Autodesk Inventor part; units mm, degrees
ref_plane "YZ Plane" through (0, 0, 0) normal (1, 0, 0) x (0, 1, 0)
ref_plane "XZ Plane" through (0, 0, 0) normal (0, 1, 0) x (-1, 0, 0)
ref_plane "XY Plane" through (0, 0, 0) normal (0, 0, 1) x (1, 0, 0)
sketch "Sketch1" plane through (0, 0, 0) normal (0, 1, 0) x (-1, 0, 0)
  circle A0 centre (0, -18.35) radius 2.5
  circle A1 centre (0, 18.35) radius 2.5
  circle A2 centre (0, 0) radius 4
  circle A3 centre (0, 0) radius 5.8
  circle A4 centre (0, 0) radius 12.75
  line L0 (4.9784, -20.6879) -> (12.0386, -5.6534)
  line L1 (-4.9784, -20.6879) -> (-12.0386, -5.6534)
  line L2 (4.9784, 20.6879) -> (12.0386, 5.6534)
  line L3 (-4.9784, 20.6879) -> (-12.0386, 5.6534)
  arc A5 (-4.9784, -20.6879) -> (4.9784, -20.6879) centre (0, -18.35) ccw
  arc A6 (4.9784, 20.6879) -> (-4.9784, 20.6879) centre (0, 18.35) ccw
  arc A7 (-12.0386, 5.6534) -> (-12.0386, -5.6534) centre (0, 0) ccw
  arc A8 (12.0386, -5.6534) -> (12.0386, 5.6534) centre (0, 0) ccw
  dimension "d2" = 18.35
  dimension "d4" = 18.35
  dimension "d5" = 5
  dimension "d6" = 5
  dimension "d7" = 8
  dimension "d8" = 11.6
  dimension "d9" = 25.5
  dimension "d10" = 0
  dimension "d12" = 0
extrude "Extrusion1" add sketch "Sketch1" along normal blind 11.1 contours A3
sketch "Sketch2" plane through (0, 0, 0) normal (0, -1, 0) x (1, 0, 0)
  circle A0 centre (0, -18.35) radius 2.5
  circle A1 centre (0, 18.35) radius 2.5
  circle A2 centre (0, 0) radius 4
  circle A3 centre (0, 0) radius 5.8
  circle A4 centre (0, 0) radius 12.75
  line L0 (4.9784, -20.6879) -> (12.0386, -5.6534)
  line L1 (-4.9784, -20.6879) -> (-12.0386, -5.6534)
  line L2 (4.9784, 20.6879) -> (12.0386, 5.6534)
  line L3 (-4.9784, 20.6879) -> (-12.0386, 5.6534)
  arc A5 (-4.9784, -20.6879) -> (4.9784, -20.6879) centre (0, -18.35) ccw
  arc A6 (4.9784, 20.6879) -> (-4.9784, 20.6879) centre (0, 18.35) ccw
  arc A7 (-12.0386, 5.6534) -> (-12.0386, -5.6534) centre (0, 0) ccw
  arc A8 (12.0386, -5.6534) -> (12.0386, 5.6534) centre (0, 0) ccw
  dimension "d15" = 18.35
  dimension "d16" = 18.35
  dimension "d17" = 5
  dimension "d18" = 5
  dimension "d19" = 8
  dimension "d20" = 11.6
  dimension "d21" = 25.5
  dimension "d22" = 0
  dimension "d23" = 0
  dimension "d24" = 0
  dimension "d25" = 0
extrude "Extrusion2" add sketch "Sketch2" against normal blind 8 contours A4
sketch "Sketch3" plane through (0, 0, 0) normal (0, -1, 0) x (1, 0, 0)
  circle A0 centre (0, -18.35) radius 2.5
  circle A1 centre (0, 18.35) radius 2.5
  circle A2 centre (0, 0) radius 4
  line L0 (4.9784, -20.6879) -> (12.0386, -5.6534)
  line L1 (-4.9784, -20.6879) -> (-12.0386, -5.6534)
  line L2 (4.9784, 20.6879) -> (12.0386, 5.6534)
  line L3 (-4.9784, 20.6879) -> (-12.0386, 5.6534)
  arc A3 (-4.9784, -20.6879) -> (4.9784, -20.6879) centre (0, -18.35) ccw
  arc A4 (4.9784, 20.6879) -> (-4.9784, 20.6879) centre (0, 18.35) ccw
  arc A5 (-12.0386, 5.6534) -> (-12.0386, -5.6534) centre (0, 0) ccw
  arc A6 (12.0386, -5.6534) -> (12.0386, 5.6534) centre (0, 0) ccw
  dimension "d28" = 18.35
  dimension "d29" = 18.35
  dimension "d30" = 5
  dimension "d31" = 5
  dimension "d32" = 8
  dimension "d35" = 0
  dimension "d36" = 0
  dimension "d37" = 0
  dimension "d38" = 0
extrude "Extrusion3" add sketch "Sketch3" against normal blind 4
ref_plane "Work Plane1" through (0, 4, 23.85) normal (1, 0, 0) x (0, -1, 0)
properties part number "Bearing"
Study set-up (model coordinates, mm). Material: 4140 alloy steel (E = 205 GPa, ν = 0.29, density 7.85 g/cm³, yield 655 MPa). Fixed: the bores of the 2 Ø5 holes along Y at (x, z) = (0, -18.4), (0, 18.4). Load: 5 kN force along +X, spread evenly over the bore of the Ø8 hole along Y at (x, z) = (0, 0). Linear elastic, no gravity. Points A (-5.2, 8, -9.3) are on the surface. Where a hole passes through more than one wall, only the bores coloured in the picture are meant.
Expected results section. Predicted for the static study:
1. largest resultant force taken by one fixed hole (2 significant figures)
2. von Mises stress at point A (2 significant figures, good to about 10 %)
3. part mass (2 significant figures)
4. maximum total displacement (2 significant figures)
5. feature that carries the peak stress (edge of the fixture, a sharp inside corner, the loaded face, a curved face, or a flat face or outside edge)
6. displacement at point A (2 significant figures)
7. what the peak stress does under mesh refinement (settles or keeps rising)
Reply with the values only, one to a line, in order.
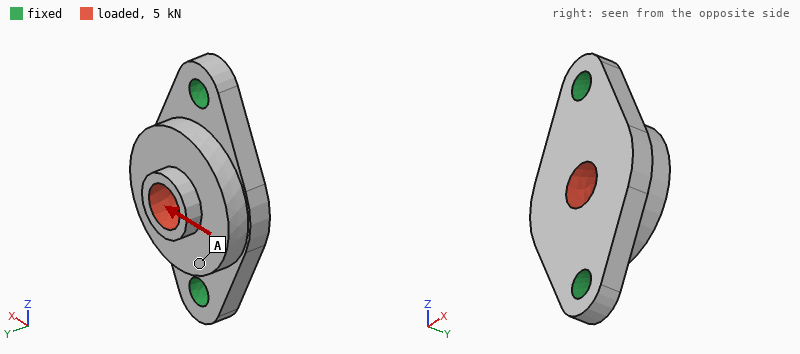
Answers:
2.5 kN
43 MPa
40 g
32 µm
edge of the fixture
20 µm
keeps rising
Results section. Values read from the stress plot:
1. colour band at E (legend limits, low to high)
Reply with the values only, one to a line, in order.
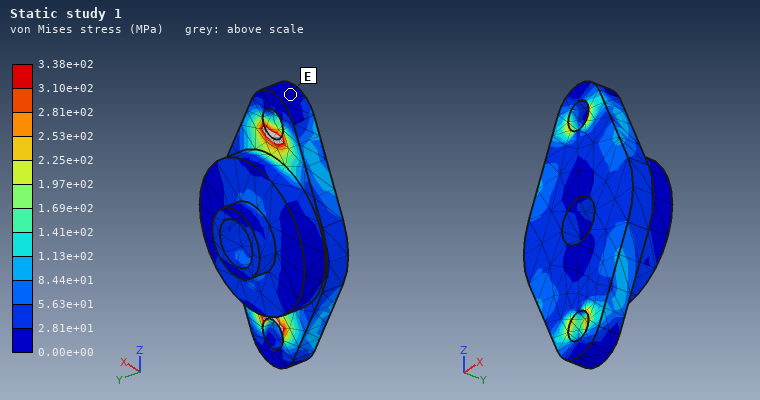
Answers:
0.00e+00 to 2.81e+01 MPa
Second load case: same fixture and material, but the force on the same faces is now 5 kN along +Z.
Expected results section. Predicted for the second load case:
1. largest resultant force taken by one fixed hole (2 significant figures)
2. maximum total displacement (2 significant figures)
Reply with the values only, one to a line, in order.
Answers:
2.6 kN
5.8 µm
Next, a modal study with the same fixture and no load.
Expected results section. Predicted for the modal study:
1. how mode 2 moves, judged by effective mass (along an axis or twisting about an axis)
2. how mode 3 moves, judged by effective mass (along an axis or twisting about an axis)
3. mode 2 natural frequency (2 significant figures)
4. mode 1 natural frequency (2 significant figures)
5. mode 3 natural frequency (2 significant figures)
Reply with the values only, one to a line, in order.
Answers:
along Y
along X
16 kHz
11 kHz
27 kHz
